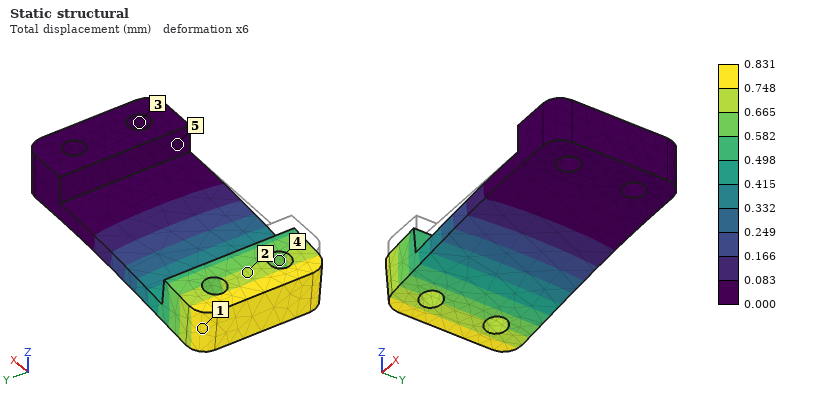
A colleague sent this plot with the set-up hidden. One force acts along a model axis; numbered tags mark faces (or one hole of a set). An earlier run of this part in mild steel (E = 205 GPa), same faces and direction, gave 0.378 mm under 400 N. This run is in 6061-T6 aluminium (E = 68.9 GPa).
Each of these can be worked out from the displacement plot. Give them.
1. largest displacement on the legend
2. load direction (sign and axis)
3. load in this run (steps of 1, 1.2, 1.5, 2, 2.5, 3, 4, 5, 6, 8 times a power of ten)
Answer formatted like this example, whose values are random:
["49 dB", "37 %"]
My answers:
["0.831 mm", "-Z", "300 N"]
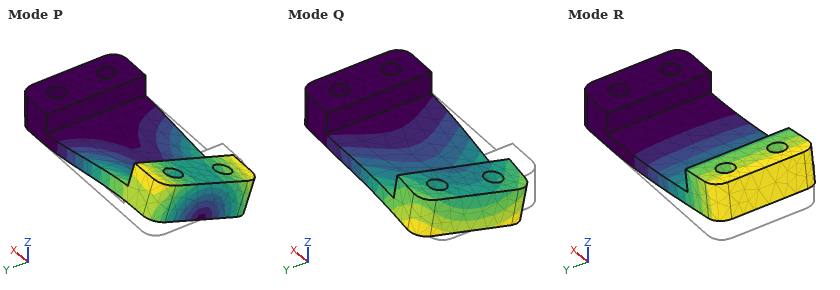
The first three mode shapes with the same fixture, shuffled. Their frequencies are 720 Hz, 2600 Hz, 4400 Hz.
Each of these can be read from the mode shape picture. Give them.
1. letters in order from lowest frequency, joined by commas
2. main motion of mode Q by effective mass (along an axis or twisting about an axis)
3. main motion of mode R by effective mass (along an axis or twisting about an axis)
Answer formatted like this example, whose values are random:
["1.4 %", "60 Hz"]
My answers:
["R, P, Q", "along Y", "along Z"]
